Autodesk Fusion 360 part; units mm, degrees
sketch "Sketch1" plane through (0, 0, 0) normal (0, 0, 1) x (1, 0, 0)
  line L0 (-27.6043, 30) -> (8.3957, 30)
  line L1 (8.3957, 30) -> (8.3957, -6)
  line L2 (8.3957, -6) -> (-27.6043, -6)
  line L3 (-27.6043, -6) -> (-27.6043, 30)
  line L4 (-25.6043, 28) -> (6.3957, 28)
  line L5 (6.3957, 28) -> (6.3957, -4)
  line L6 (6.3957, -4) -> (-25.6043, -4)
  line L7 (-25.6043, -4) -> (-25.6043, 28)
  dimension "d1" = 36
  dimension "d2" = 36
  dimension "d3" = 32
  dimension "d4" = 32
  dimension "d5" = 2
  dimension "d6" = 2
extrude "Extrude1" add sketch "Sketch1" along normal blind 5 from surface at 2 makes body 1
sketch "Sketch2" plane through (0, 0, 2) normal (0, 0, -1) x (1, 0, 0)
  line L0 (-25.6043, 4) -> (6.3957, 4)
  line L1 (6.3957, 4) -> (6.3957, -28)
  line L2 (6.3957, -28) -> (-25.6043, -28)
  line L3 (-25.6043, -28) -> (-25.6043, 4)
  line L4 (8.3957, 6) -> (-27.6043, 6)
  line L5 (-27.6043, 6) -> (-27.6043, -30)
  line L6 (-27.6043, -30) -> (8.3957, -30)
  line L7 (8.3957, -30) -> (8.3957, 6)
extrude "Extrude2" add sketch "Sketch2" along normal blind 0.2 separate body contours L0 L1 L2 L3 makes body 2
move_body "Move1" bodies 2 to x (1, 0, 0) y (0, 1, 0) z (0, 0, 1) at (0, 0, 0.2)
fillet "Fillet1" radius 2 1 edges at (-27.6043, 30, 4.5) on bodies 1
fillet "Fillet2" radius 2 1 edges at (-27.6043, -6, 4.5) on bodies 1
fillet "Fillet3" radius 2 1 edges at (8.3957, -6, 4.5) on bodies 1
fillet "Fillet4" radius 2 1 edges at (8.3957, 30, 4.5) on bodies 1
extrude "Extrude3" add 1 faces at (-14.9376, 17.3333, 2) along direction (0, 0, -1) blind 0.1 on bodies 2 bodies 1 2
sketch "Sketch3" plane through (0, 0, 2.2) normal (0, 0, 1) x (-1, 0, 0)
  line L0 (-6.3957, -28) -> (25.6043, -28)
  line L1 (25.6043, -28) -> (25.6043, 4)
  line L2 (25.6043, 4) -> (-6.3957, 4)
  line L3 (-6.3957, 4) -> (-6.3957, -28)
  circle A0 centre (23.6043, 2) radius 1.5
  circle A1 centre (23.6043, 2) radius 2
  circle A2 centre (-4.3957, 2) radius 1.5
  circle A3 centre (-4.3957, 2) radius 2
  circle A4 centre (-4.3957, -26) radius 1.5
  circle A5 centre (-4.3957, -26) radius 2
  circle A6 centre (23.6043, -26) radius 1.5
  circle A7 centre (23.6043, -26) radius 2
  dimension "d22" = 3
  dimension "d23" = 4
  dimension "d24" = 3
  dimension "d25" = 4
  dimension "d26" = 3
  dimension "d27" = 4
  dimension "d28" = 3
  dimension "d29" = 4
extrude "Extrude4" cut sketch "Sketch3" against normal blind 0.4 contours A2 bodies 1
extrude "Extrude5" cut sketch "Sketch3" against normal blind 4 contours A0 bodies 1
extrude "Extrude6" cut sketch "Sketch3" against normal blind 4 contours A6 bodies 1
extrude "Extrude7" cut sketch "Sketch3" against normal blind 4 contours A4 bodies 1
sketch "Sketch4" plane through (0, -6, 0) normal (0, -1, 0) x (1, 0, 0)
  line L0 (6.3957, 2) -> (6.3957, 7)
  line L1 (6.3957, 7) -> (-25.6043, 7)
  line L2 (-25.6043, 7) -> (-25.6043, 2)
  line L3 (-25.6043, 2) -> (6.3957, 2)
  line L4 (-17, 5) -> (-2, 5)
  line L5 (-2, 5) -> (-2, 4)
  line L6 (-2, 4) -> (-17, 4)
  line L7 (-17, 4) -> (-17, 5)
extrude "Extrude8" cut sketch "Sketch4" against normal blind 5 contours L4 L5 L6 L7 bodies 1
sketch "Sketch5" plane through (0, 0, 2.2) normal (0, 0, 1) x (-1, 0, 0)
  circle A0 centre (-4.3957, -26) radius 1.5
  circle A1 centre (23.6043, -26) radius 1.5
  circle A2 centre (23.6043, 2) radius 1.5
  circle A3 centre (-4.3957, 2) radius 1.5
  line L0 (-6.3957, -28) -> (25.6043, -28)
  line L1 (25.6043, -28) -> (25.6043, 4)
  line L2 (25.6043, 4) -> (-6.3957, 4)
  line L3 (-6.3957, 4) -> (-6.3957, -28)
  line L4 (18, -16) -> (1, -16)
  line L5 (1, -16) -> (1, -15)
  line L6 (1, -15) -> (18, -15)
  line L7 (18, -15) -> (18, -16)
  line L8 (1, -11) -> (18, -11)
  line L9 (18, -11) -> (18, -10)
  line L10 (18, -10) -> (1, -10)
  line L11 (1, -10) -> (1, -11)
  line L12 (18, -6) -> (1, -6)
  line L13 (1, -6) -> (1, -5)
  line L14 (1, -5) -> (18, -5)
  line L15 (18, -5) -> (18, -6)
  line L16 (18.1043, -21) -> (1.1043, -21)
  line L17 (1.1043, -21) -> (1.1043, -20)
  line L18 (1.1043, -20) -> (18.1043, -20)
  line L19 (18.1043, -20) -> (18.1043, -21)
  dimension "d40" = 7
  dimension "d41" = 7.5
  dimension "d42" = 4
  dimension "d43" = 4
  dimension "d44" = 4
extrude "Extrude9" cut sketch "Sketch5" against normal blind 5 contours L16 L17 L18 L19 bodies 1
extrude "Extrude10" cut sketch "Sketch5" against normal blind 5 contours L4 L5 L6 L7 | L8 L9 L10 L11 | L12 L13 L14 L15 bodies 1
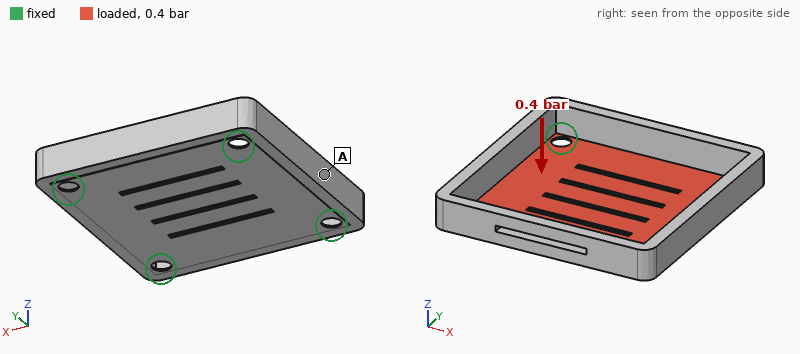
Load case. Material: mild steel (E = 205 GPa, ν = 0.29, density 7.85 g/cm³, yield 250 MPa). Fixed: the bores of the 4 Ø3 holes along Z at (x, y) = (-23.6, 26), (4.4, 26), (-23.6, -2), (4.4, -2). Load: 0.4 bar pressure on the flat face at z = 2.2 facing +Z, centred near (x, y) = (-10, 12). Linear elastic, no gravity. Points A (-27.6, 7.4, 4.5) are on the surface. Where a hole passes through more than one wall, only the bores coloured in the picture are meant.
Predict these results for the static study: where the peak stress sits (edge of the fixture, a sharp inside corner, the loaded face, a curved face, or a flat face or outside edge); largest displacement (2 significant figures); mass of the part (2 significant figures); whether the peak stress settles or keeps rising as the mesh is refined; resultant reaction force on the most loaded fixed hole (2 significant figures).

a sharp inside corner
0.17 mm
12 g
keeps rising
14 N
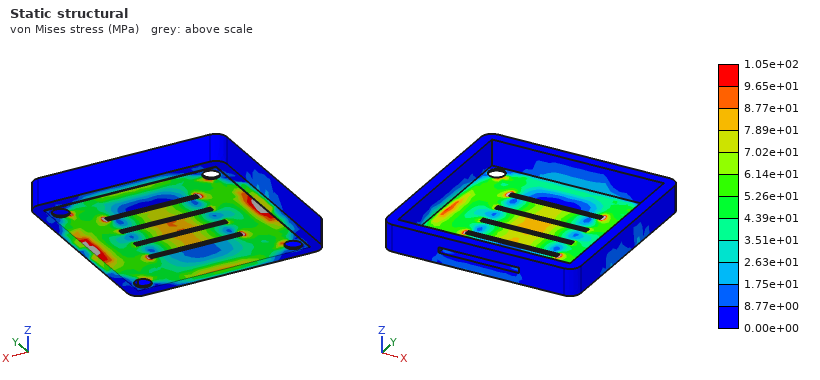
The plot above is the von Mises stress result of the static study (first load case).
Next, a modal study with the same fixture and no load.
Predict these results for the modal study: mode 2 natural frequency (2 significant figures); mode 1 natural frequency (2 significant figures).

3000 Hz
2100 Hz
